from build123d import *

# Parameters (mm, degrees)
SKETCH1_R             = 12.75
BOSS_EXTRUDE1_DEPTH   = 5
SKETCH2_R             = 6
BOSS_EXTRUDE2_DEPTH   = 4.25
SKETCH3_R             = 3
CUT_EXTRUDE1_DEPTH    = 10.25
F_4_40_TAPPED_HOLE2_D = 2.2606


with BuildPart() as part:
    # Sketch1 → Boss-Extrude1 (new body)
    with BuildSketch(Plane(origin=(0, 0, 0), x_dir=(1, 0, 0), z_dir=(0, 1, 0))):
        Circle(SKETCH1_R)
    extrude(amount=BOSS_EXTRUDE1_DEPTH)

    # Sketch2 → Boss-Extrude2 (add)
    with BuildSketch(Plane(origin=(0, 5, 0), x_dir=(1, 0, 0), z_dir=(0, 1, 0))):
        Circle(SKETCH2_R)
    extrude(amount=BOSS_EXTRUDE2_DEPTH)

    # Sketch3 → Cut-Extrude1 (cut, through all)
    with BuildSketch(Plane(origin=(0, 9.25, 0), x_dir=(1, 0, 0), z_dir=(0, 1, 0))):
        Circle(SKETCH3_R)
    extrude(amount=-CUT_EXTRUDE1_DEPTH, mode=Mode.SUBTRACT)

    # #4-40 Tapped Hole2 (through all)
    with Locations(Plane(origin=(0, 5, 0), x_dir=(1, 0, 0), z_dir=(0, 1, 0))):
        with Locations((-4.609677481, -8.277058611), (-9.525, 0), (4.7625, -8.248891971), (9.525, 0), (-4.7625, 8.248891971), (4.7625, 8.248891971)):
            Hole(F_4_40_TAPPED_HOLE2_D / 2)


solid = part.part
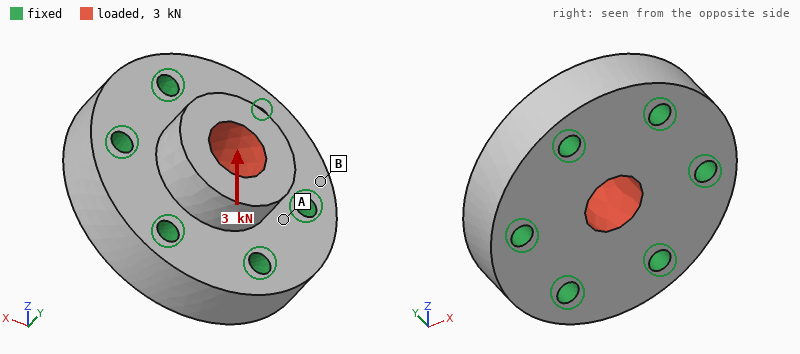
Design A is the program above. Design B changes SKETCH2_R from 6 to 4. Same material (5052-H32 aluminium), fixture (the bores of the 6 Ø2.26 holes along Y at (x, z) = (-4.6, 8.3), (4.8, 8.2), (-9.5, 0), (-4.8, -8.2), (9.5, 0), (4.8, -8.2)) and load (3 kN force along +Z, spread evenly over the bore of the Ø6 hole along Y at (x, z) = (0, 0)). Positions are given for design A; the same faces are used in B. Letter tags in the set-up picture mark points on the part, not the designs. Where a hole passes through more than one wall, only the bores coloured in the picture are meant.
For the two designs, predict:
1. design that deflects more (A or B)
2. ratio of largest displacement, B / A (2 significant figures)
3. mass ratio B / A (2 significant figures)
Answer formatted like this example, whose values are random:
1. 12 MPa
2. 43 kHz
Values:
1. B
2. 3.2
3. 0.90
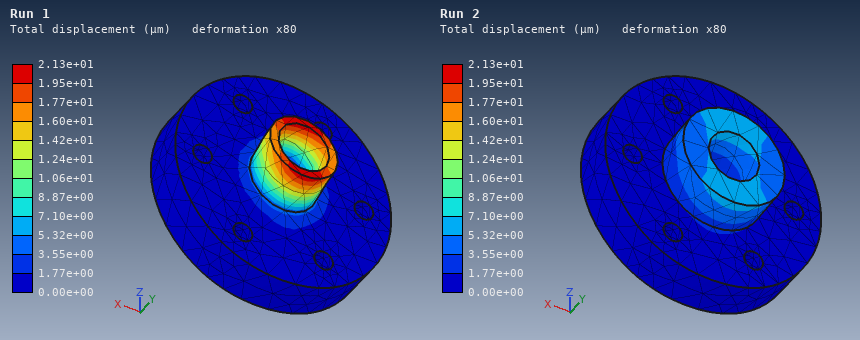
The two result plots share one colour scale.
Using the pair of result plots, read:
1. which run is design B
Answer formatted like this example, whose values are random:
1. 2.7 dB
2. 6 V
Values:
1. Run 1
